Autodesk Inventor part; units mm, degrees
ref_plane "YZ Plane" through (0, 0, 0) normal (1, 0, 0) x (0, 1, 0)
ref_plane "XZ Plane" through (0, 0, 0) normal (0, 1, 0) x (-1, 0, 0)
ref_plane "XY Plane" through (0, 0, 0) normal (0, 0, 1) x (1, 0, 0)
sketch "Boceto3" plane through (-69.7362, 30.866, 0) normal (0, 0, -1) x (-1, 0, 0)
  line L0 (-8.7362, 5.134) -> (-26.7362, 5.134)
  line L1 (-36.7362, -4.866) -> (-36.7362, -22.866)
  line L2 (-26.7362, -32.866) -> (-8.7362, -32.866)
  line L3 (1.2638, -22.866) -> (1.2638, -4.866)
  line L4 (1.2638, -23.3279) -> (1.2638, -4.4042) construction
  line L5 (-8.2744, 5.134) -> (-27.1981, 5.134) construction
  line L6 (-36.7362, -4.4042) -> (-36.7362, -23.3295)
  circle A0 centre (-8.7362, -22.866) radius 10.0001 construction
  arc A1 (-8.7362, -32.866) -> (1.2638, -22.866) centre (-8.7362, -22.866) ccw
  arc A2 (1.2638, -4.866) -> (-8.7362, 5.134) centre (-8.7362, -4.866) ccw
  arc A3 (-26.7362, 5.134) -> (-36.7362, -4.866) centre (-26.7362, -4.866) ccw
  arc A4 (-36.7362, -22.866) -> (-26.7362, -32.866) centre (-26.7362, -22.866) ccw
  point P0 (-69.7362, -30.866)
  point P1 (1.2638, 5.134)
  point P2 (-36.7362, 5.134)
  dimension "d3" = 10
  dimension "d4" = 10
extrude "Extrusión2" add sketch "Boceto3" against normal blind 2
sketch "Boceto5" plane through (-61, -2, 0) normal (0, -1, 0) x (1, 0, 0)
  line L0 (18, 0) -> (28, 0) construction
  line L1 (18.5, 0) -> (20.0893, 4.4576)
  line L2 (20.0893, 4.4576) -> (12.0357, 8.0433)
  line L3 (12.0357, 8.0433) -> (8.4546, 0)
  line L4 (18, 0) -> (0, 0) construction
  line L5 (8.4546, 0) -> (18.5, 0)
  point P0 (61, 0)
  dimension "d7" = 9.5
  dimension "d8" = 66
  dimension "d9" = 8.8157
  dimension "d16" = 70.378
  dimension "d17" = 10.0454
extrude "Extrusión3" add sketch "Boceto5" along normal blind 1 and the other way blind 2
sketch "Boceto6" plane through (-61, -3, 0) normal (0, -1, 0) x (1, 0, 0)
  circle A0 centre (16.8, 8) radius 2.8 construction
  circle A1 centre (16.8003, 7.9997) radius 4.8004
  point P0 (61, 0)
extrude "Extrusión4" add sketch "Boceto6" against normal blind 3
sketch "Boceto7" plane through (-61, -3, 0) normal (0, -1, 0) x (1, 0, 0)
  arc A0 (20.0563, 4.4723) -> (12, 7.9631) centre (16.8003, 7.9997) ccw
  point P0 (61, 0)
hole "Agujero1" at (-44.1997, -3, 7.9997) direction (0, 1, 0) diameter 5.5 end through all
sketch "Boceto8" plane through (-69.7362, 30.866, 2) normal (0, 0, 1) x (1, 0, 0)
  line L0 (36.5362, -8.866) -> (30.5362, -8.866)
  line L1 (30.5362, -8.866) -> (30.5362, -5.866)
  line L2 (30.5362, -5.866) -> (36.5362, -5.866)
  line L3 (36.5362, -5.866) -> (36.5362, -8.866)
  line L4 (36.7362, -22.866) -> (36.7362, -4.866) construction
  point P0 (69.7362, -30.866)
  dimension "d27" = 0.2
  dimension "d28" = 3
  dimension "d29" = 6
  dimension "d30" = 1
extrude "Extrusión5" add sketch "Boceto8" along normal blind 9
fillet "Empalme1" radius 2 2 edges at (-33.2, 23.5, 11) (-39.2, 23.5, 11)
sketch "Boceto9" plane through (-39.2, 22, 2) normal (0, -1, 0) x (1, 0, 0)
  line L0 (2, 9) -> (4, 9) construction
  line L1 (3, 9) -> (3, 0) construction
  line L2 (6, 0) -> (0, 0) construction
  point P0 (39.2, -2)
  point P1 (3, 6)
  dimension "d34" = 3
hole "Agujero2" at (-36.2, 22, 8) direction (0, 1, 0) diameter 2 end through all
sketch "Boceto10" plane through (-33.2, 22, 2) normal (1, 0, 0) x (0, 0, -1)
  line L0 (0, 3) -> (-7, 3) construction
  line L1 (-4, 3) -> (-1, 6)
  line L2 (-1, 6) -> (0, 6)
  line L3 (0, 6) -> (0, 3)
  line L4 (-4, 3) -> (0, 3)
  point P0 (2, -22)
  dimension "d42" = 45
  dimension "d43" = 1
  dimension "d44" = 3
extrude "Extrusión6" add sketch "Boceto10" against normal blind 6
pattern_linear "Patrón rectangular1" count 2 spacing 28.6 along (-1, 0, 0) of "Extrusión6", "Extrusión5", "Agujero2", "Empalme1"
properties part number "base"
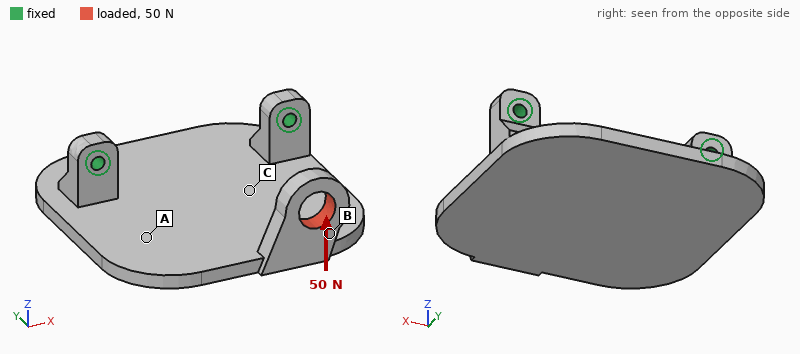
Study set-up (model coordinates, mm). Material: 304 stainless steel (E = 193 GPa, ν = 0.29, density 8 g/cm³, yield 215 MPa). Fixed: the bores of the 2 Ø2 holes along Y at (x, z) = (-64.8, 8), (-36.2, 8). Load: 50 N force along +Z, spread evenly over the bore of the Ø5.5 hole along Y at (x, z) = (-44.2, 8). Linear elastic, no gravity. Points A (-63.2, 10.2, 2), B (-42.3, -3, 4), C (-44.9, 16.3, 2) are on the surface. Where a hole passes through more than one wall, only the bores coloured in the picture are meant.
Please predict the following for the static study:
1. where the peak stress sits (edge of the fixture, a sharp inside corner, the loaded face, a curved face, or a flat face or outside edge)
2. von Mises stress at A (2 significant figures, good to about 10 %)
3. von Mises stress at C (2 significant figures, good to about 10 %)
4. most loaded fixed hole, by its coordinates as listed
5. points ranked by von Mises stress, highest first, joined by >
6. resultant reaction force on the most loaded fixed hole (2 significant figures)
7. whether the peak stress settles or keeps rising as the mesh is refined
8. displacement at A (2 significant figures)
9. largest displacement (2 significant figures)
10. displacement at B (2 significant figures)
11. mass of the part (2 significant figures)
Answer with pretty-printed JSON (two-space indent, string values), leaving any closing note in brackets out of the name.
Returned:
{
  "where the peak stress sits": "edge of the fixture",
  "von Mises stress at A": "22 MPa",
  "von Mises stress at C": "36 MPa",
  "most loaded fixed hole, by its coordinates as listed": "(-36.2, 8)",
  "points ranked by von Mises stress, highest first, joined by >": "C > A > B",
  "resultant reaction force on the most loaded fixed hole": "42 N",
  "whether the peak stress settles or keeps rising as the mesh is refined": "keeps rising",
  "displacement at A": "0.029 mm",
  "largest displacement": "0.11 mm",
  "displacement at B": "0.099 mm",
  "mass of the part": "27 g"
}
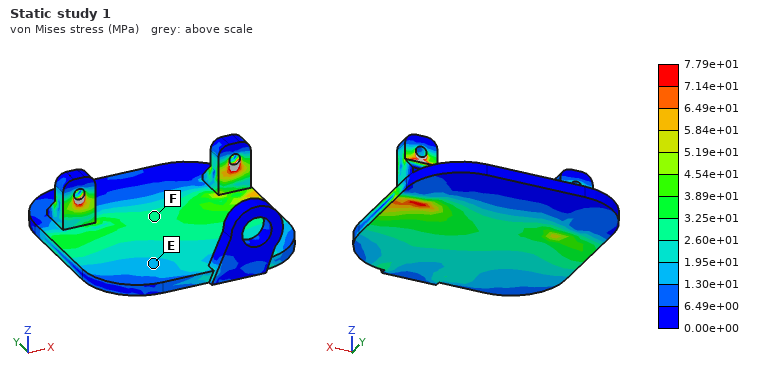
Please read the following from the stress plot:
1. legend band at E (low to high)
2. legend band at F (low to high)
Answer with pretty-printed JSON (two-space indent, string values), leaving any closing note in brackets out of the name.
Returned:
{
  "legend band at E": "1.30e+01 to 1.95e+01 MPa",
  "legend band at F": "2.60e+01 to 3.25e+01 MPa"
}
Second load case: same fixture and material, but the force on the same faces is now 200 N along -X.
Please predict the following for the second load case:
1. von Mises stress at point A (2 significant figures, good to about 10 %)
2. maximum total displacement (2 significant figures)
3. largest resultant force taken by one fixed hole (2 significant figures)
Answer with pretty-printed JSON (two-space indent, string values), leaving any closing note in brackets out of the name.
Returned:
{
  "von Mises stress at point A": "28 MPa",
  "maximum total displacement": "87 µm",
  "largest resultant force taken by one fixed hole": "190 N"
}
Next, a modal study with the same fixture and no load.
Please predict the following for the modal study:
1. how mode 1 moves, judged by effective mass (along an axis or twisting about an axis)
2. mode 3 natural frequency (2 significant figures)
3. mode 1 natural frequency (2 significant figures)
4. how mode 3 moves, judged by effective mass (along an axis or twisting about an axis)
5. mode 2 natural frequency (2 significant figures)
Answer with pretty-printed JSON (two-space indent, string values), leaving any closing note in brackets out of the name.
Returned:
{
  "how mode 1 moves, judged by effective mass": "along Z",
  "mode 3 natural frequency": "6100 Hz",
  "mode 1 natural frequency": "1600 Hz",
  "how mode 3 moves, judged by effective mass": "along Y",
  "mode 2 natural frequency": "4100 Hz"
}
